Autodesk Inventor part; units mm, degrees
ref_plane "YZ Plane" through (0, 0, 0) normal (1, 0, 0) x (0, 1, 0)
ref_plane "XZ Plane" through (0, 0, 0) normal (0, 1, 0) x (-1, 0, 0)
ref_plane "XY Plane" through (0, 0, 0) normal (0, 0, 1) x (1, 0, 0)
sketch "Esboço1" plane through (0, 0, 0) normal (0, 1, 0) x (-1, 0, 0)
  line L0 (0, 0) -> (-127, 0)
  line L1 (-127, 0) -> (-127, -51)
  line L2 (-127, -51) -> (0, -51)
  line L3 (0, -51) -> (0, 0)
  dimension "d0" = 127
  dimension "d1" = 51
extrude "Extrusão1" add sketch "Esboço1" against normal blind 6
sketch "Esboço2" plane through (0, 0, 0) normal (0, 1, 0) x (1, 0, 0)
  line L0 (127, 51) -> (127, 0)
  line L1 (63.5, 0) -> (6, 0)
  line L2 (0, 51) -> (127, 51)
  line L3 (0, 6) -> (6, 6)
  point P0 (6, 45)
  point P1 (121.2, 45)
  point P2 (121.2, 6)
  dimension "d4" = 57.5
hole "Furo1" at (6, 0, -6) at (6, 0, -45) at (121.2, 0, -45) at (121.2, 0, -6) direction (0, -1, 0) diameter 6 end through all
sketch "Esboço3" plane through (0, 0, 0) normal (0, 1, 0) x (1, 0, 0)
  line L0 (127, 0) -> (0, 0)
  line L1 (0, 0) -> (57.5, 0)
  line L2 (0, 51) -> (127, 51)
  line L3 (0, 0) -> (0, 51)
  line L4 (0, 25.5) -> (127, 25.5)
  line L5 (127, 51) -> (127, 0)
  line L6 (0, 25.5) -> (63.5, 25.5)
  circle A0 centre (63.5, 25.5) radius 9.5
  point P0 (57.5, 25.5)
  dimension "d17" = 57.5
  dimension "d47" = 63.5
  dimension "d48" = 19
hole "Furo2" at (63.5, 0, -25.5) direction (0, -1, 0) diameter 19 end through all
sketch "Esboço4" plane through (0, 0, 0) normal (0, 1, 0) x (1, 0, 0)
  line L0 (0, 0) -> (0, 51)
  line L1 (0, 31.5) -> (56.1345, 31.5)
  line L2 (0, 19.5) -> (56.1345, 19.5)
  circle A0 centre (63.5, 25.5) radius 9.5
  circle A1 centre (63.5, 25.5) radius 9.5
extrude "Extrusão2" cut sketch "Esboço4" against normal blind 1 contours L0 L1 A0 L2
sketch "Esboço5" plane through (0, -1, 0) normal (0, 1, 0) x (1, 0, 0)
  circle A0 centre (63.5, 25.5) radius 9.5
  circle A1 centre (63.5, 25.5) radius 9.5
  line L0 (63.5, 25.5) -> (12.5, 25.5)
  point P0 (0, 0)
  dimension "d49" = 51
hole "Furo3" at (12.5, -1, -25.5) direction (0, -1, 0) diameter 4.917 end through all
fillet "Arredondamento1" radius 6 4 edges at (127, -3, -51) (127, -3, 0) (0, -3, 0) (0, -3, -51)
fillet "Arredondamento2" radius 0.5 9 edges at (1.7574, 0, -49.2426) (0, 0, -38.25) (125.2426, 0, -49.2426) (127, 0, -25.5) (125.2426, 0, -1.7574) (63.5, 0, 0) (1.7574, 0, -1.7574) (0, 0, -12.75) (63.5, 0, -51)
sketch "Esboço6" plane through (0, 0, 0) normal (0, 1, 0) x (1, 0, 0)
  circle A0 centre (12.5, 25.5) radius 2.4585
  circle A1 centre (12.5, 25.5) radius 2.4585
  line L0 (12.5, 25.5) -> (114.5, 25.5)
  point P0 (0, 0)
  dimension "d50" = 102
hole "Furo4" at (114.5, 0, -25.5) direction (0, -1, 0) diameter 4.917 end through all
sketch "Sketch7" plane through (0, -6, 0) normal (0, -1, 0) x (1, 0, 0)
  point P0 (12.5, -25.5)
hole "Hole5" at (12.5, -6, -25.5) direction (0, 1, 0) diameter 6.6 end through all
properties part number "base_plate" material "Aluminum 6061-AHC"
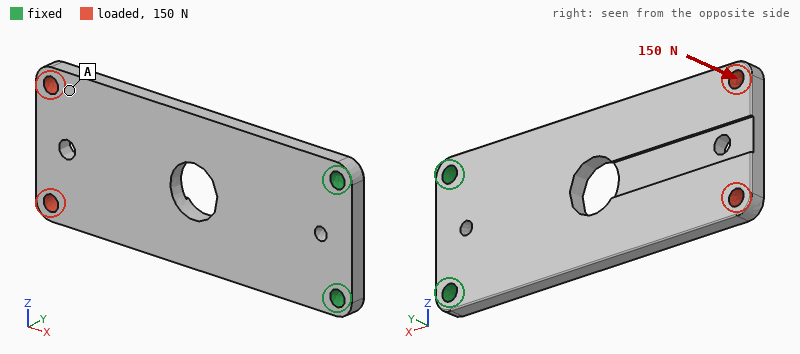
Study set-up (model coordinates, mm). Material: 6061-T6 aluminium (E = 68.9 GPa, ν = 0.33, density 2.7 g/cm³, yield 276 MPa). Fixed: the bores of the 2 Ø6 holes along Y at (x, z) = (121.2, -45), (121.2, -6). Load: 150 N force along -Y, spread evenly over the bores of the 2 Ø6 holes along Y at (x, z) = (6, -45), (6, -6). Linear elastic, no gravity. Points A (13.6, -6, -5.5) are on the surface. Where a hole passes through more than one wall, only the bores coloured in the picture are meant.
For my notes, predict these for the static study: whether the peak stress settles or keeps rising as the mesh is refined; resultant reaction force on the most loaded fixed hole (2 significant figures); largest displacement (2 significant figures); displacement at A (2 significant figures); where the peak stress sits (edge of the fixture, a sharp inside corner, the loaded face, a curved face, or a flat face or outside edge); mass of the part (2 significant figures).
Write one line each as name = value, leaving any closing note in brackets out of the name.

whether the peak stress settles or keeps rising as the mesh is refined = keeps rising
resultant reaction force on the most loaded fixed hole = 75 N
largest displacement = 1.5 mm
displacement at A = 1.2 mm
where the peak stress sits = edge of the fixture
mass of the part = 95 g
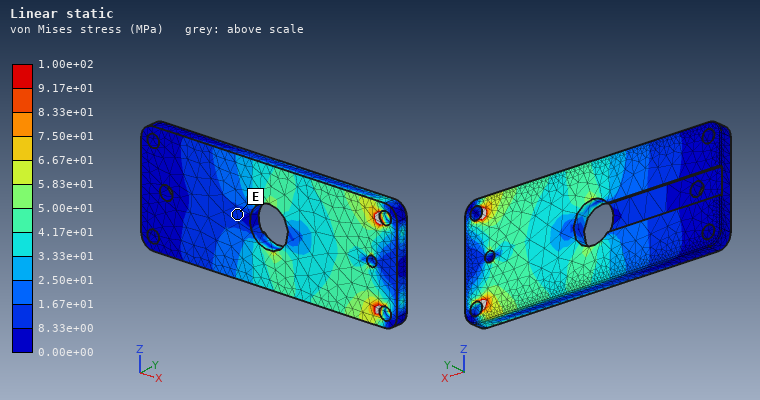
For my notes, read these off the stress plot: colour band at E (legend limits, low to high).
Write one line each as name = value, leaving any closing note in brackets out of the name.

colour band at E = 8.33e+00 to 1.67e+01 MPa
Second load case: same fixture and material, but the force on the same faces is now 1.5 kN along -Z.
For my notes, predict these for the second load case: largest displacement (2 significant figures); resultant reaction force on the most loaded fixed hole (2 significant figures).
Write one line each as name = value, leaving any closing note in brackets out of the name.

largest displacement = 0.22 mm
resultant reaction force on the most loaded fixed hole = 4.3 kN
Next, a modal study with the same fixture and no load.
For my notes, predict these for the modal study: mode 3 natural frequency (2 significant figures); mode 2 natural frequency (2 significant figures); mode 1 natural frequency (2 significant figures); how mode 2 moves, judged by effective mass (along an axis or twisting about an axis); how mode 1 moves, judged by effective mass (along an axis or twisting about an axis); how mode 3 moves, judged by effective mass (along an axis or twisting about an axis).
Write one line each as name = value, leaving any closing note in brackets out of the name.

mode 3 natural frequency = 2000 Hz
mode 2 natural frequency = 1600 Hz
mode 1 natural frequency = 340 Hz
how mode 2 moves, judged by effective mass = twisting about X
how mode 1 moves, judged by effective mass = along Y
how mode 3 moves, judged by effective mass = along Y
